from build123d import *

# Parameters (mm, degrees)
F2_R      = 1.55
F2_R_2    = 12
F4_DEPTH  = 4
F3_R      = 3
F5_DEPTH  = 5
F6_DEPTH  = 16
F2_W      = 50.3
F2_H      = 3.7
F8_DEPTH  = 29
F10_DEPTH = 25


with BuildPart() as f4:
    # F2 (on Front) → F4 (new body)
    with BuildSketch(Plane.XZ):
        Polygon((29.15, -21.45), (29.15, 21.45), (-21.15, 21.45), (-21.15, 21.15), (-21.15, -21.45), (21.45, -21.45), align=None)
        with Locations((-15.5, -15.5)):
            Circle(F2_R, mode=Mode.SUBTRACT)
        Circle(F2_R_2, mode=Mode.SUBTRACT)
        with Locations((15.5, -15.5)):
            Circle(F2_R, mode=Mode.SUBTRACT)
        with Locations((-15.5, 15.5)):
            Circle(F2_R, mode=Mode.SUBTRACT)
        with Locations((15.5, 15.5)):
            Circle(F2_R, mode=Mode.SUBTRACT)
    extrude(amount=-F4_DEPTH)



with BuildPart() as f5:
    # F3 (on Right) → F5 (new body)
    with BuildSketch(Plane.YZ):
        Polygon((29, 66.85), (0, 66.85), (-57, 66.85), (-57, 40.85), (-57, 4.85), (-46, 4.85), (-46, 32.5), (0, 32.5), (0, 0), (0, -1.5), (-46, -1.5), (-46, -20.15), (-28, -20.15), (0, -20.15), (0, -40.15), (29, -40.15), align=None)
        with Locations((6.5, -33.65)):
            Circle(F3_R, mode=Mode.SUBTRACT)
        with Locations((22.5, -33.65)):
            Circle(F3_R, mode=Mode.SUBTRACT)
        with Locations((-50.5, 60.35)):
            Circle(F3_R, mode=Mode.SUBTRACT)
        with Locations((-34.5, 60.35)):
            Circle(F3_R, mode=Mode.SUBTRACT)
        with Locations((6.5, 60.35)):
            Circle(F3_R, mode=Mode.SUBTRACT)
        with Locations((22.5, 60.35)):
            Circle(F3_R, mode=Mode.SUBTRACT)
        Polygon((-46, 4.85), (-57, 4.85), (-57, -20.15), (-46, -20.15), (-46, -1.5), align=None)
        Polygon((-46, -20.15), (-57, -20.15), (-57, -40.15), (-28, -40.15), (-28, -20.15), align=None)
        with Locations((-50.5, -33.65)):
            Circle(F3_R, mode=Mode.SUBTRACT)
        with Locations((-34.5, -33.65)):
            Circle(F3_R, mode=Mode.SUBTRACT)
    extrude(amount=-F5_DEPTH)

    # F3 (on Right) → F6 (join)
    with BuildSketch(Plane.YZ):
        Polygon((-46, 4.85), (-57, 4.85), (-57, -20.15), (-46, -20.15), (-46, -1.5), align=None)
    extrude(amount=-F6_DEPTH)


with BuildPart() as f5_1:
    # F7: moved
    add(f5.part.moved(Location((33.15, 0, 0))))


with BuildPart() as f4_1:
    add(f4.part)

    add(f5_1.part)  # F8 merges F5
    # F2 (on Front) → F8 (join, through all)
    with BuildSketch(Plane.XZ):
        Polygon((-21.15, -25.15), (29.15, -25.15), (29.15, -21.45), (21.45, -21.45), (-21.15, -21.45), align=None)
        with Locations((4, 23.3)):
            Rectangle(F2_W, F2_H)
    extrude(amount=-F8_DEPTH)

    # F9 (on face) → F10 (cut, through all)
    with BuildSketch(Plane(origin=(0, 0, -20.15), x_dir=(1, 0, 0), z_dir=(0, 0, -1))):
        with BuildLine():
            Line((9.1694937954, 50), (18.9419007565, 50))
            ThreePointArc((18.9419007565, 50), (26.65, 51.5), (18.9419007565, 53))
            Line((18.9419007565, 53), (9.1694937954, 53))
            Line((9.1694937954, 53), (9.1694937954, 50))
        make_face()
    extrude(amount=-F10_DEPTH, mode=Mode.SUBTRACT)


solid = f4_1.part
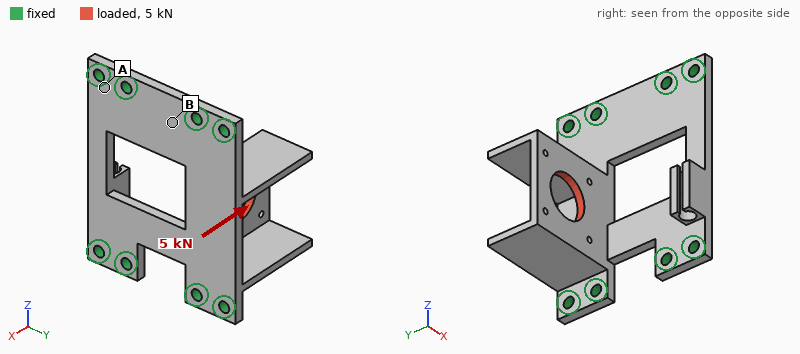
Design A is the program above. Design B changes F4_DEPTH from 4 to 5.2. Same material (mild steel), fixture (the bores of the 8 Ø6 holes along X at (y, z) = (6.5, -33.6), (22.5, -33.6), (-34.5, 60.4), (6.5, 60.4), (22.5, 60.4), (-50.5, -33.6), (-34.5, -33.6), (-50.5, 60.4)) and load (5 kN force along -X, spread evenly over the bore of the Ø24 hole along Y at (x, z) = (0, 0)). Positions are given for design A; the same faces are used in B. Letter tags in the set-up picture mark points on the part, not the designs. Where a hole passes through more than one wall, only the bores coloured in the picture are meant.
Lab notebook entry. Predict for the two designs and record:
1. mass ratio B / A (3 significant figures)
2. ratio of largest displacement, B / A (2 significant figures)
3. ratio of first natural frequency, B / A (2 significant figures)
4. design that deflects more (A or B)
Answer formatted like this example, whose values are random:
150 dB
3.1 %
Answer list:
1.04
0.92
1.0
A
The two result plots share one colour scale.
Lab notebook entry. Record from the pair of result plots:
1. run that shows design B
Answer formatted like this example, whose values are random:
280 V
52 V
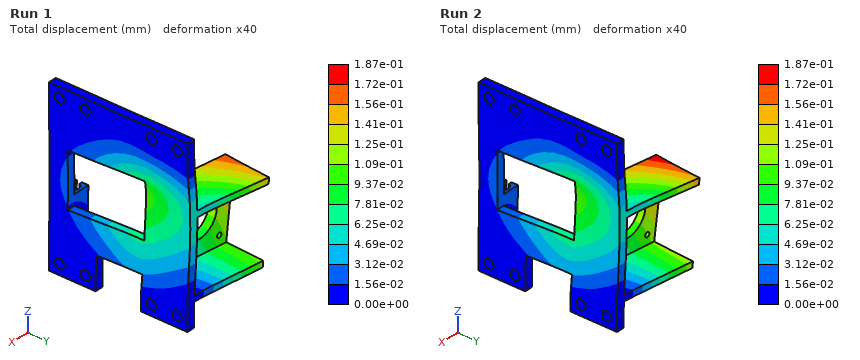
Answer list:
Run 1
